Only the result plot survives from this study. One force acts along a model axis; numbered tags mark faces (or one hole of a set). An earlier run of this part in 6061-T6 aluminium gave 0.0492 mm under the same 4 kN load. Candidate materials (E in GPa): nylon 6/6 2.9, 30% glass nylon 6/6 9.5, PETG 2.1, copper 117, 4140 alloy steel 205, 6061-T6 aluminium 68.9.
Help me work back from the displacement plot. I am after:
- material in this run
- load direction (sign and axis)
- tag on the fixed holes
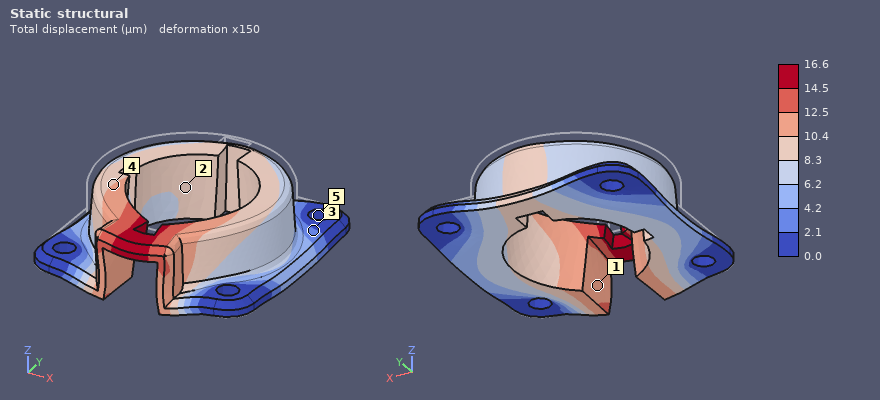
4140 alloy steel
-Z
5
